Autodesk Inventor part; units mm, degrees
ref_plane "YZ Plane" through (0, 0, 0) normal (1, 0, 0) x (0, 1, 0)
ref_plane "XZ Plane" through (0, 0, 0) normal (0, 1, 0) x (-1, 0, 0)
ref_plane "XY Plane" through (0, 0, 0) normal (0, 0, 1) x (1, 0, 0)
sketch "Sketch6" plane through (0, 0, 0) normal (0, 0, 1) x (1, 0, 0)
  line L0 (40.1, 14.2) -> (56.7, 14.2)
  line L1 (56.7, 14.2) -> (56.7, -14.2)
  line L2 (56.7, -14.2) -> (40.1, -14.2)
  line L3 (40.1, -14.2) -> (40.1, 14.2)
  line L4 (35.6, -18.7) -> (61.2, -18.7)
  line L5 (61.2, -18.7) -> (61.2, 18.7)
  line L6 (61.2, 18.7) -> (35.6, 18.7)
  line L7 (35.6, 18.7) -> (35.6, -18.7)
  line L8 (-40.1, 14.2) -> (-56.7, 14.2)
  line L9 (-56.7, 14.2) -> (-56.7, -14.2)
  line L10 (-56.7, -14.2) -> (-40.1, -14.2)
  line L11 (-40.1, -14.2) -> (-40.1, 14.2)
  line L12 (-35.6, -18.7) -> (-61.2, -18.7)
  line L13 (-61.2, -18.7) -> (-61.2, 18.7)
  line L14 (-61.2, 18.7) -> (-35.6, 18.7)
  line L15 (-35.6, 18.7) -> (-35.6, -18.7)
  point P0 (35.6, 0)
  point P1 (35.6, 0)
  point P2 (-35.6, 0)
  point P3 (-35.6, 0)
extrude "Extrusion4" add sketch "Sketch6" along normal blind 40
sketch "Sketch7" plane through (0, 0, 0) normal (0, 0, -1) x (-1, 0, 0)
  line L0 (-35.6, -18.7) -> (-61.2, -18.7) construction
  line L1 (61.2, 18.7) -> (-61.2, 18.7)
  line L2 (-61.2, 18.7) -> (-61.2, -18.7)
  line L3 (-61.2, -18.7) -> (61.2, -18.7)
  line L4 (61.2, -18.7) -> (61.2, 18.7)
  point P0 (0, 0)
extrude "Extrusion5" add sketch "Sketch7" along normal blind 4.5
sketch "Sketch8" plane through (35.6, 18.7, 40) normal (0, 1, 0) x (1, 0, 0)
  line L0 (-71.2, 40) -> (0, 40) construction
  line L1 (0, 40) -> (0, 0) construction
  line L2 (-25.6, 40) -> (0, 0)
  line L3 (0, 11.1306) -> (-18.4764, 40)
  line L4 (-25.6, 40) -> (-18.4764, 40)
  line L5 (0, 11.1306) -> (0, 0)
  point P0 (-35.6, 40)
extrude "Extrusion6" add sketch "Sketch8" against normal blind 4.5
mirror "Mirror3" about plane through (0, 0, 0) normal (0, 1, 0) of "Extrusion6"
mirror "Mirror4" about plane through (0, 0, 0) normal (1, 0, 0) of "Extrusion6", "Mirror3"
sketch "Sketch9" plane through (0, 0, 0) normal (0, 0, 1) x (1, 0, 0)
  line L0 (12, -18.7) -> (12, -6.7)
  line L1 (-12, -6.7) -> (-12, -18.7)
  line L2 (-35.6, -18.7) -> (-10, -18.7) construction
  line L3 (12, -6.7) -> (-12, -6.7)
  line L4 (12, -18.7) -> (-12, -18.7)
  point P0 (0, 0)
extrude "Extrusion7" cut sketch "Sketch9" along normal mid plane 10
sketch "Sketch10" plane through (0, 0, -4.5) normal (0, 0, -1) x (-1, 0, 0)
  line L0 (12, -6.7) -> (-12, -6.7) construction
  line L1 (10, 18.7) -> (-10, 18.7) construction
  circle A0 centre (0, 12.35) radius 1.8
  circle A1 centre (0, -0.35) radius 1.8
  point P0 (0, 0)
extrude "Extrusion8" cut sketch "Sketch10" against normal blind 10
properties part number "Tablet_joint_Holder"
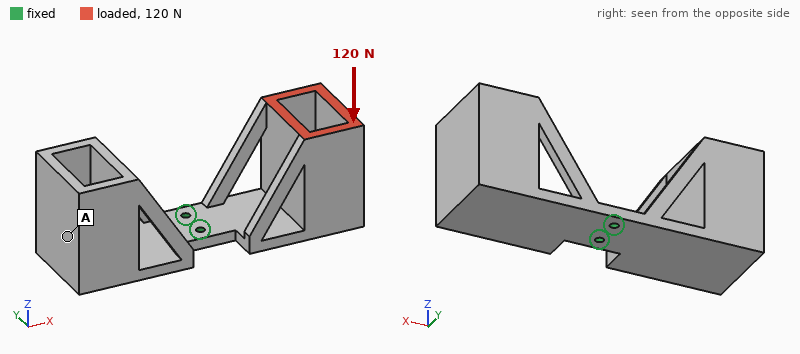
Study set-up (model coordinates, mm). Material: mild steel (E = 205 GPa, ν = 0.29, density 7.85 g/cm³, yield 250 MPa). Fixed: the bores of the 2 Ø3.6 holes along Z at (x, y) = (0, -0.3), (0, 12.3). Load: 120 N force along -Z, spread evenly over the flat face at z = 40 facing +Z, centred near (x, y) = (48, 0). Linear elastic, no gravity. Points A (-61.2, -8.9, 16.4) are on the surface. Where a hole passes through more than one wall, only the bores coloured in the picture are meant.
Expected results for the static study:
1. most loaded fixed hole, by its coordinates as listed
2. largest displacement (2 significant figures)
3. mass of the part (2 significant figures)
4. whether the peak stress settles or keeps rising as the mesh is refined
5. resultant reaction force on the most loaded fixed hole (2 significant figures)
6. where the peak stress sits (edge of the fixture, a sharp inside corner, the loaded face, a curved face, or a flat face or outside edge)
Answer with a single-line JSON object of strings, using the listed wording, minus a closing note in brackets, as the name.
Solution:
{"most loaded fixed hole, by its coordinates as listed": "(0, -0.3)", "largest displacement": "0.14 mm", "mass of the part": "490 g", "whether the peak stress settles or keeps rising as the mesh is refined": "keeps rising", "resultant reaction force on the most loaded fixed hole": "100 N", "where the peak stress sits": "edge of the fixture"}
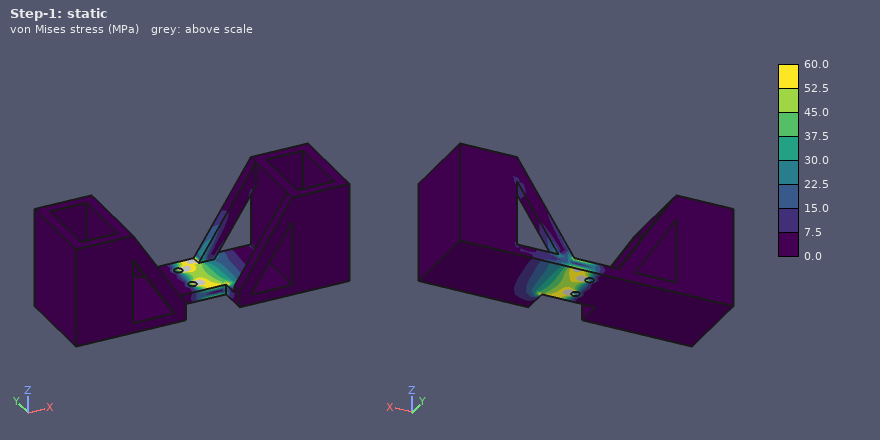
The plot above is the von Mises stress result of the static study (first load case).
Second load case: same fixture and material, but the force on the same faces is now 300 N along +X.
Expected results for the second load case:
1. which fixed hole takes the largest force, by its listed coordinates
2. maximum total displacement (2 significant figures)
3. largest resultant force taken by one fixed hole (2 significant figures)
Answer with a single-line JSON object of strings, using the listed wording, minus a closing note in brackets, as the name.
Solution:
{"which fixed hole takes the largest force, by its listed coordinates": "(0, -0.3)", "maximum total displacement": "0.39 mm", "largest resultant force taken by one fixed hole": "280 N"}
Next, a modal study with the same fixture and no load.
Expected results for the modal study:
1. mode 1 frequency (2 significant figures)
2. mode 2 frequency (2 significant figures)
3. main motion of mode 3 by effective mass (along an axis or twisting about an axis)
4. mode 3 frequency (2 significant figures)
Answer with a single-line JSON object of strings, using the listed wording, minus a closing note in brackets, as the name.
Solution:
{"mode 1 frequency": "360 Hz", "mode 2 frequency": "380 Hz", "main motion of mode 3 by effective mass": "twisting about Z", "mode 3 frequency": "860 Hz"}
